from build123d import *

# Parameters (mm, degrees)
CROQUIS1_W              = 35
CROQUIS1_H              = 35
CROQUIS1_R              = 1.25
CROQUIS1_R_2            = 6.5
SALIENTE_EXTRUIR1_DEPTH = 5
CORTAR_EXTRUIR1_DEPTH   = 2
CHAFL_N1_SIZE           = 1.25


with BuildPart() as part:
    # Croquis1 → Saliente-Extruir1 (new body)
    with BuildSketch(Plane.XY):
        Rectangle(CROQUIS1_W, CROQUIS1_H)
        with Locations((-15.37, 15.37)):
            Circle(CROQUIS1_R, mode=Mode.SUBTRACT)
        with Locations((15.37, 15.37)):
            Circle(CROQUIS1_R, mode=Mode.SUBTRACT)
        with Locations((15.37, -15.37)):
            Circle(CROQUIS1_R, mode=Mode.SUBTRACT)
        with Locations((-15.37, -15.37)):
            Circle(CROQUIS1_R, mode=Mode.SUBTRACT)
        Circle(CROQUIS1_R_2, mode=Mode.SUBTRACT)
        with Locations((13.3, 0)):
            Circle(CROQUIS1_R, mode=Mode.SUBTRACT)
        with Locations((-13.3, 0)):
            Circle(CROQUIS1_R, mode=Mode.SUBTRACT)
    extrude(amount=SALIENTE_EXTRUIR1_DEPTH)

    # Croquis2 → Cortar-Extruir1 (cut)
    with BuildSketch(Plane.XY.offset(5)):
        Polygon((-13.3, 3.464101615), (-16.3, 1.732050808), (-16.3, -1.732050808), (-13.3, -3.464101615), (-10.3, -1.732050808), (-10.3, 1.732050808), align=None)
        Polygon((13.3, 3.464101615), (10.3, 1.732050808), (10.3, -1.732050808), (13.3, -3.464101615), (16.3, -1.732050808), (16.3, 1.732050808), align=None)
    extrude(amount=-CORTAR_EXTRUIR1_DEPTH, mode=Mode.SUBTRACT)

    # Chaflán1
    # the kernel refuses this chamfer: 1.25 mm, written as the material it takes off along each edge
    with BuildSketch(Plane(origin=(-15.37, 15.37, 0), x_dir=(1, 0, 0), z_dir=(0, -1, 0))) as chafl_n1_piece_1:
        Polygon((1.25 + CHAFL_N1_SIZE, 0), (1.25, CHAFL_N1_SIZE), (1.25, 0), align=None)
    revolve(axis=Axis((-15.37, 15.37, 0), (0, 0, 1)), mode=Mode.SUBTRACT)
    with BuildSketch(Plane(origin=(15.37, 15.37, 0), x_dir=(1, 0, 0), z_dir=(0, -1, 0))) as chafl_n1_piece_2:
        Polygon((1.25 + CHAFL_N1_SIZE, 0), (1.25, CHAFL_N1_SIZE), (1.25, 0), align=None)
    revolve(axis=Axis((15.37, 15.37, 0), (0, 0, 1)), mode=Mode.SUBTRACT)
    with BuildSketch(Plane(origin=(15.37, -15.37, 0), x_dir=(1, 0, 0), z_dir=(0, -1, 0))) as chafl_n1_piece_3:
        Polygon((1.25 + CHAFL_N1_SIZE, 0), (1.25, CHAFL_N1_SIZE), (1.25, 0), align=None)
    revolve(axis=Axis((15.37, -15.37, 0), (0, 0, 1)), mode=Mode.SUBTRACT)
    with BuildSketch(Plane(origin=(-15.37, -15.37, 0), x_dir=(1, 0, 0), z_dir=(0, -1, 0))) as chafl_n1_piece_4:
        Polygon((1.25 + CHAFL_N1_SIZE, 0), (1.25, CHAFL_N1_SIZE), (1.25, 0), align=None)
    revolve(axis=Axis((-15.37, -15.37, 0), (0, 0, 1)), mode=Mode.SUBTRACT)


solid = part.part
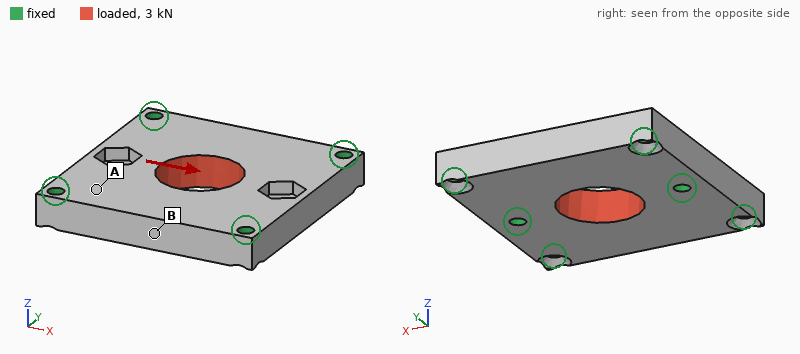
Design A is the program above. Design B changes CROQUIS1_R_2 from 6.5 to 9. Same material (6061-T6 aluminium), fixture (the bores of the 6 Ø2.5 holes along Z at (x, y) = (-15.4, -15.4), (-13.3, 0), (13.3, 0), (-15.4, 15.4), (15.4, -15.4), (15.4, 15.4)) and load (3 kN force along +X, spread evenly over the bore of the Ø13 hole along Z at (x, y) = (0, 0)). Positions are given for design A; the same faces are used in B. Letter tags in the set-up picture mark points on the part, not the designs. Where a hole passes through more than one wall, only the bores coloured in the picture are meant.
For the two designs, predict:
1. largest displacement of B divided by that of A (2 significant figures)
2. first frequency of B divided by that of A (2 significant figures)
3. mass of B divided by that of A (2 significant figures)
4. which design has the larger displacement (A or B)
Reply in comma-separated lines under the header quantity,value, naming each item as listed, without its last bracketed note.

quantity,value
largest displacement of B divided by that of A,1.2
first frequency of B divided by that of A,1.0
mass of B divided by that of A,0.88
which design has the larger displacement,B
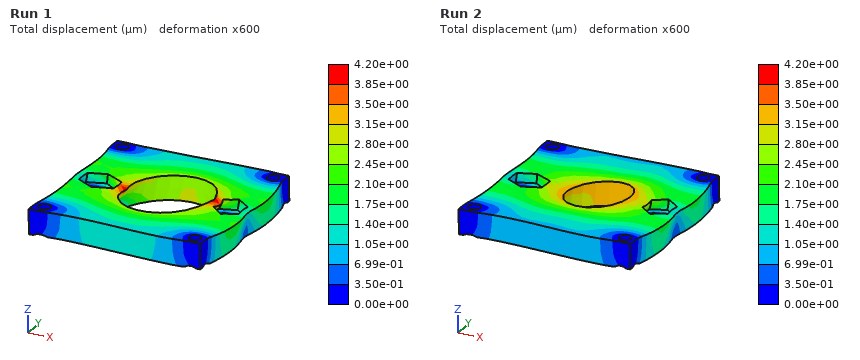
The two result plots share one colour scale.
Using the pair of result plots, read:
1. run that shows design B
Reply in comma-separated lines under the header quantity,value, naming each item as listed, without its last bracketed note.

quantity,value
run that shows design B,Run 1
